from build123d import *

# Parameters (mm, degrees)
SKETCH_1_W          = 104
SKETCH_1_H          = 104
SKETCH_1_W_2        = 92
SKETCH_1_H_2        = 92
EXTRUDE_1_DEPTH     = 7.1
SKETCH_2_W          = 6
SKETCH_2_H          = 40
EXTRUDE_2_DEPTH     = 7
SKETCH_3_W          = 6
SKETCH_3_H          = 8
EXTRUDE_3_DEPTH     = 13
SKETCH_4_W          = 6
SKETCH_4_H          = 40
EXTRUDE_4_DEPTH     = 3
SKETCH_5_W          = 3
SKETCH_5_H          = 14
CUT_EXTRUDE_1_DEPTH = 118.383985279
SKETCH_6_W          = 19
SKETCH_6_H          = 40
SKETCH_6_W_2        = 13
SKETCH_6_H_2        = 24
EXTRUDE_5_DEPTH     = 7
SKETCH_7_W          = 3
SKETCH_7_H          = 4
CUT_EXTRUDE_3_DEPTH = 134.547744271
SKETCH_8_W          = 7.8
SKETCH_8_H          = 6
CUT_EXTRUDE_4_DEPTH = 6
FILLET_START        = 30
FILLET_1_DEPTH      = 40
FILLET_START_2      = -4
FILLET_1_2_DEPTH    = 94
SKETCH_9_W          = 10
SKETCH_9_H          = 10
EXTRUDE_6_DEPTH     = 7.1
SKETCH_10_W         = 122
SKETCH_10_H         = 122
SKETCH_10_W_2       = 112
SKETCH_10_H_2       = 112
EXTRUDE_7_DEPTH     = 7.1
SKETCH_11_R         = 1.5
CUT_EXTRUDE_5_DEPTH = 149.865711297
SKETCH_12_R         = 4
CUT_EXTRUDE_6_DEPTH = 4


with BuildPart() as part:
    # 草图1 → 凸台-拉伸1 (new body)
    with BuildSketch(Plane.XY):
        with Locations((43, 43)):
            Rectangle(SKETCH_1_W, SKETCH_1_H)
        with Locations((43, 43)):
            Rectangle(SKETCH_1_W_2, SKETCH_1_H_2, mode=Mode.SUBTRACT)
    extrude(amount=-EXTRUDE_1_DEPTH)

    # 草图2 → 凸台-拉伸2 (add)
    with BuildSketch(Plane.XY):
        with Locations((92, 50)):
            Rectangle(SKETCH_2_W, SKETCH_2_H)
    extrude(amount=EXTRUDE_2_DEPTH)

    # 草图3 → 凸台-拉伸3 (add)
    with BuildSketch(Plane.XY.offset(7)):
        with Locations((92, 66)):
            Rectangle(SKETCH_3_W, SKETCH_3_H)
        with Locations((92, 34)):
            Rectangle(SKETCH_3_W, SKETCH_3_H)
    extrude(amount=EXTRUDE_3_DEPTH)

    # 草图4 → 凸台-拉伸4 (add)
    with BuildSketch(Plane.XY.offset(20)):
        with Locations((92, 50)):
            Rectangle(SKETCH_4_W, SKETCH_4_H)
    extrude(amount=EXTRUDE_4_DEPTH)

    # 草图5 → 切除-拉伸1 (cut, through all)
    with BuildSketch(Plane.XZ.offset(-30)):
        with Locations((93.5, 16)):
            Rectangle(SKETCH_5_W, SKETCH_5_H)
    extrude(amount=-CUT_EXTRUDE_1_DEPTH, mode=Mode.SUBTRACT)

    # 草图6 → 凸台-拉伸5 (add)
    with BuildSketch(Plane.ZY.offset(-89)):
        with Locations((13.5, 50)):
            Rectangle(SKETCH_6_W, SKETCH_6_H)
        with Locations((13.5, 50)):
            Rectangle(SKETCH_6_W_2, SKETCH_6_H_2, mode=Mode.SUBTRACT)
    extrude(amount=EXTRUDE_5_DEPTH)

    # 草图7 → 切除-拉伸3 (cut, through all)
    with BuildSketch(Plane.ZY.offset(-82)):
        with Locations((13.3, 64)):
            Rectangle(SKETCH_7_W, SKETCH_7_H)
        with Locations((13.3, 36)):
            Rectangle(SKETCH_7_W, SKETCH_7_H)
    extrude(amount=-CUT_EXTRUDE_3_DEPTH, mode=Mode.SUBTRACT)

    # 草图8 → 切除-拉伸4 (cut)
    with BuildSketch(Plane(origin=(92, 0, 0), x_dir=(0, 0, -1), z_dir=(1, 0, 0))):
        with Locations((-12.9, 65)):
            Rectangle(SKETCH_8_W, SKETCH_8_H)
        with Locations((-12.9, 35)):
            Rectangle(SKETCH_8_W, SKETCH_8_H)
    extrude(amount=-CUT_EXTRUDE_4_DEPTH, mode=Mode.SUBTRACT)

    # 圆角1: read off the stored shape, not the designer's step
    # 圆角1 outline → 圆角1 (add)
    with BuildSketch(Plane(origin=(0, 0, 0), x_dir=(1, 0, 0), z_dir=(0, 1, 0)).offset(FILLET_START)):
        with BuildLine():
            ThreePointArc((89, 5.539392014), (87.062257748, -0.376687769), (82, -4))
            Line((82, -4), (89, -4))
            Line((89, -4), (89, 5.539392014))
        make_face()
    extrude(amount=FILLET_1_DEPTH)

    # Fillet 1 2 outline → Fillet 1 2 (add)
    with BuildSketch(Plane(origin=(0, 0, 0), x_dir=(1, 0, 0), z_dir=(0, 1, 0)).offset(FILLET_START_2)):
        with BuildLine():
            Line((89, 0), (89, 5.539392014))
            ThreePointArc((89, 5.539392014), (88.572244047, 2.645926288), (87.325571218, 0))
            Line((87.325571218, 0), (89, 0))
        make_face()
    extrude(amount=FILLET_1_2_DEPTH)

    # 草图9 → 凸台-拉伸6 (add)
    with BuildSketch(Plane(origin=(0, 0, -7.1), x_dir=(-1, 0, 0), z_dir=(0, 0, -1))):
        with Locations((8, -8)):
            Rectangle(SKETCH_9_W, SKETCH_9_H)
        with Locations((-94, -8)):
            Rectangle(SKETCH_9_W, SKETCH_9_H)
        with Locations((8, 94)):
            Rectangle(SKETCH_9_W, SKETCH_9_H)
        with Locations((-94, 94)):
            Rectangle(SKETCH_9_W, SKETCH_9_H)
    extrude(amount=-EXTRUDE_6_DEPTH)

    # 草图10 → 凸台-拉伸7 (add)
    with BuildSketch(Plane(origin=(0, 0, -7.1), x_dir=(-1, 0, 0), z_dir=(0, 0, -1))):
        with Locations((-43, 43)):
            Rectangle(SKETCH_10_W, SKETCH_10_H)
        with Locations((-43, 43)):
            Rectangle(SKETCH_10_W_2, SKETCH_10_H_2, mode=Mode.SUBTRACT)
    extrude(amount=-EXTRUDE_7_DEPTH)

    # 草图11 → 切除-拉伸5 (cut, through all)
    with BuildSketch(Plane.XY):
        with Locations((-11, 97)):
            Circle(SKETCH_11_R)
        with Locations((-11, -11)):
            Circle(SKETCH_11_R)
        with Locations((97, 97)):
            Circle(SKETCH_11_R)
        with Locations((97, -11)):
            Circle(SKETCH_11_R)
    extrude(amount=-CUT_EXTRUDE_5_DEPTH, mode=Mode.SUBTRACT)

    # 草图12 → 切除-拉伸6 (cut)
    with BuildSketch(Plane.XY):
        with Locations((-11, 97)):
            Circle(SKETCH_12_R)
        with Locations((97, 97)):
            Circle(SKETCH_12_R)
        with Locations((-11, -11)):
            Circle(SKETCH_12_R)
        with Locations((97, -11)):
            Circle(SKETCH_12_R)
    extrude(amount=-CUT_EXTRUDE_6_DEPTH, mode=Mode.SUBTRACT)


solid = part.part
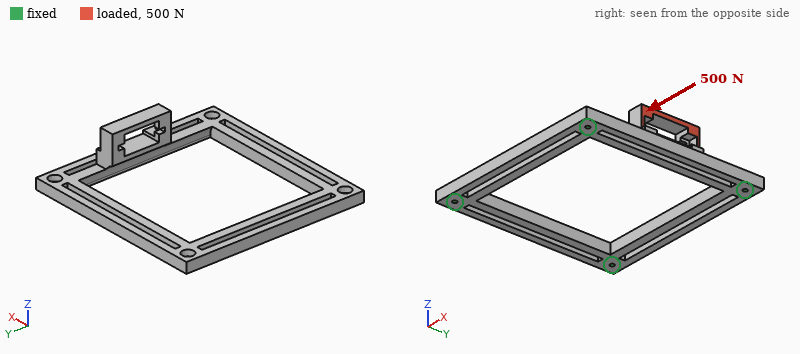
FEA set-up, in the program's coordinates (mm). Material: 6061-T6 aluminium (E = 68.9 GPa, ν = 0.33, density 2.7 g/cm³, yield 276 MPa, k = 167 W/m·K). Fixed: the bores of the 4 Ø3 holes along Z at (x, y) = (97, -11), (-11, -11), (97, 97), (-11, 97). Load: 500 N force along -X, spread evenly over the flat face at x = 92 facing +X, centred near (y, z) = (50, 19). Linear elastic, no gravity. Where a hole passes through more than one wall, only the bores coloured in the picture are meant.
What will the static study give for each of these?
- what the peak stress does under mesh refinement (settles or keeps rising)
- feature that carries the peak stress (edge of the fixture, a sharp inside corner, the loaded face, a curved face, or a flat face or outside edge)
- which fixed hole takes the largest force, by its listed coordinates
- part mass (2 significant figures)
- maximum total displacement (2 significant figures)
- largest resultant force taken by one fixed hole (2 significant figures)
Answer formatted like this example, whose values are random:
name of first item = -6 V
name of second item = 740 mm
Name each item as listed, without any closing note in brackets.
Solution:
what the peak stress does under mesh refinement = keeps rising
feature that carries the peak stress = edge of the fixture
which fixed hole takes the largest force, by its listed coordinates = (-11, 97)
part mass = 110 g
maximum total displacement = 0.88 mm
largest resultant force taken by one fixed hole = 330 N
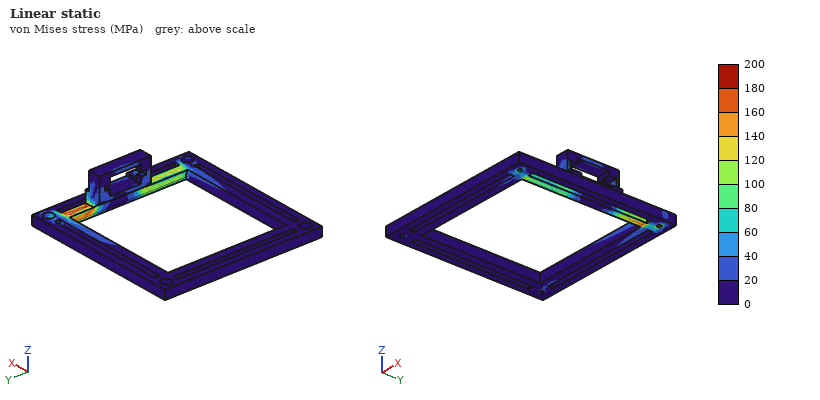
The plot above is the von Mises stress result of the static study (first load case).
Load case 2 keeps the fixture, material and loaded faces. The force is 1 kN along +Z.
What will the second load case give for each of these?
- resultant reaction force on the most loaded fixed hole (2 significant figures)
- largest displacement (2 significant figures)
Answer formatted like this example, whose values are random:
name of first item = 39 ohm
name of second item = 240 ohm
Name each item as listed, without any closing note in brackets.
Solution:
resultant reaction force on the most loaded fixed hole = 1.1 kN
largest displacement = 0.31 mm
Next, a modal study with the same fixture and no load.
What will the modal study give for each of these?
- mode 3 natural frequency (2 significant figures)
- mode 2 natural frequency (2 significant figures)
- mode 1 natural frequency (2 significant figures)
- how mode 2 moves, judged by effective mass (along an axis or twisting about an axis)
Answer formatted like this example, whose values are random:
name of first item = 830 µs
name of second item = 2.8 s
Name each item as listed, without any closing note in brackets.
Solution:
mode 3 natural frequency = 2400 Hz
mode 2 natural frequency = 2100 Hz
mode 1 natural frequency = 1400 Hz
how mode 2 moves, judged by effective mass = along Z
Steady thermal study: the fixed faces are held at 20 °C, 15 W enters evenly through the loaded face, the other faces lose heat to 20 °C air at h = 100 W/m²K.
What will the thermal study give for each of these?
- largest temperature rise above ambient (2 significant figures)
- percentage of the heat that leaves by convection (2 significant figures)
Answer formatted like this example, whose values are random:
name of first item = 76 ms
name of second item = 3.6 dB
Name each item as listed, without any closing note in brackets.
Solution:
largest temperature rise above ambient = 33 K
percentage of the heat that leaves by convection = 67 %
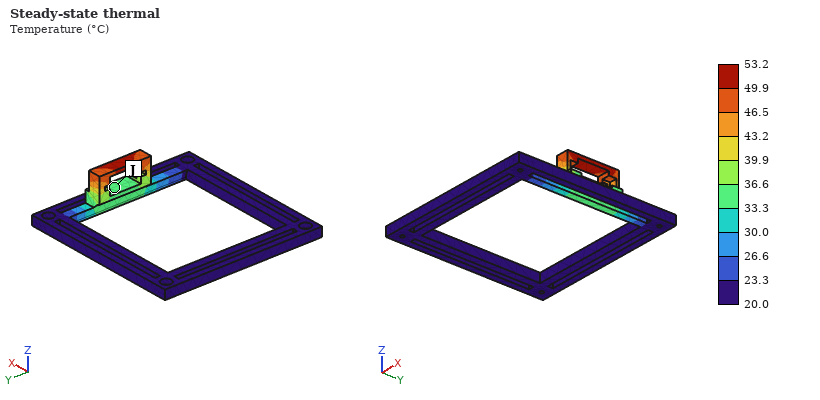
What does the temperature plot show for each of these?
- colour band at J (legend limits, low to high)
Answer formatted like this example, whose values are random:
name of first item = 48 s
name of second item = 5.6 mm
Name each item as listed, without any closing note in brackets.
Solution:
colour band at J = 33.3 to 36.6 °C
